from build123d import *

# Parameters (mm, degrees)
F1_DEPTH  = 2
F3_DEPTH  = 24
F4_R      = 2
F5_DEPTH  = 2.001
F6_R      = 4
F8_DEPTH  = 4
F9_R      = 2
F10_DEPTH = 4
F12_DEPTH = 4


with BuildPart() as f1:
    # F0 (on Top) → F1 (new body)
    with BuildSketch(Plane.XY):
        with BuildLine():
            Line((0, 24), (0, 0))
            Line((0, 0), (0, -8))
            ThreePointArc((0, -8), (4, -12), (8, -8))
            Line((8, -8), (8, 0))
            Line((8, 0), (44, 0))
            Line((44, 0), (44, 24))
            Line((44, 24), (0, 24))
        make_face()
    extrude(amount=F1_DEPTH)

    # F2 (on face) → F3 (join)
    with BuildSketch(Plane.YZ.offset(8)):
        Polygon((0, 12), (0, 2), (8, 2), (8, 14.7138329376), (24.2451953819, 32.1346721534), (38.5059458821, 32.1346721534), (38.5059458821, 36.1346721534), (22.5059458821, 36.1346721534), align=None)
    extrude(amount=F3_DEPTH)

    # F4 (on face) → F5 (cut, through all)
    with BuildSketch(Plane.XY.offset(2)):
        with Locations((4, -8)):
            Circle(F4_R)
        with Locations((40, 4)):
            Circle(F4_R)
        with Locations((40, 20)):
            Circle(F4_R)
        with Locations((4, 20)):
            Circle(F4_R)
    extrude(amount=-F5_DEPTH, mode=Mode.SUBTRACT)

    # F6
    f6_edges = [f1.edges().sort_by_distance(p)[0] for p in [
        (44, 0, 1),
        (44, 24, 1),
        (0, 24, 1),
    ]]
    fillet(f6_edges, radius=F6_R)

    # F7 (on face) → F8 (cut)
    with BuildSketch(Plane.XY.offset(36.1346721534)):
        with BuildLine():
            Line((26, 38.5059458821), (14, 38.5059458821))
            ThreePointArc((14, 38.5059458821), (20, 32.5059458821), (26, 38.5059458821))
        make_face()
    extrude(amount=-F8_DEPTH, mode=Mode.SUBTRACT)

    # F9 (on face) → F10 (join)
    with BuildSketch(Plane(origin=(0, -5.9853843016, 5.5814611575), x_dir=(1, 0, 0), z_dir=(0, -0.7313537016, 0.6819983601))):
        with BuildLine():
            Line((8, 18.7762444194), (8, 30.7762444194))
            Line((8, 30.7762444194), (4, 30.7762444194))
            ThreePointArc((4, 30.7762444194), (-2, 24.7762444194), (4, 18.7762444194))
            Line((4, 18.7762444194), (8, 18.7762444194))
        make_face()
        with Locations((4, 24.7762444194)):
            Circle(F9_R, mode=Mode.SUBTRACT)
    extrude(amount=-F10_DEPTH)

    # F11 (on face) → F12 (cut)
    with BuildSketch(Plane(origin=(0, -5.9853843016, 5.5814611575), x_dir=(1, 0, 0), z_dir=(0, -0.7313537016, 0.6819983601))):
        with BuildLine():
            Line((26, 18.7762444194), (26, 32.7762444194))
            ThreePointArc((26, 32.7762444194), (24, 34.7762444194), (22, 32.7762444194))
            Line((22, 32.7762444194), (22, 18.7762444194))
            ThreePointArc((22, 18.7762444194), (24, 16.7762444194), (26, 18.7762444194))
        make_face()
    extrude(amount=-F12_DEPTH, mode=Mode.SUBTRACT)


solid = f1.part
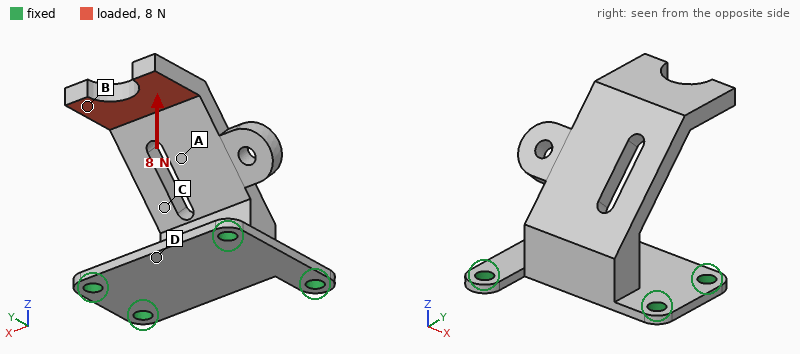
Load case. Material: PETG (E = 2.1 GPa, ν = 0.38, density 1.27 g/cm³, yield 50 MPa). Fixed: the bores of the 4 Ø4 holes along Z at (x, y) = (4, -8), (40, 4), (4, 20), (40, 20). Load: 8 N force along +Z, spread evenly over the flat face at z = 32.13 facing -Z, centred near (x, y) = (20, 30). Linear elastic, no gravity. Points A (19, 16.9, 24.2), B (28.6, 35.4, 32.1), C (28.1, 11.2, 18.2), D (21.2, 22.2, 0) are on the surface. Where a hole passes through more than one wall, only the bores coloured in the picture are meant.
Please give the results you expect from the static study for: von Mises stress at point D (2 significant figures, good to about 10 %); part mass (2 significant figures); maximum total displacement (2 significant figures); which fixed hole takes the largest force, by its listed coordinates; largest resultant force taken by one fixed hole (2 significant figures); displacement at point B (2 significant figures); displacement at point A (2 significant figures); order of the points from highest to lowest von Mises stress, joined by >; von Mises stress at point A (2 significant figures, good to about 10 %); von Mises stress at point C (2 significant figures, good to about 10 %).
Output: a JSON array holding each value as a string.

["1.3 MPa", "11 g", "0.89 mm", "(4, 20)", "8.4 N", "0.77 mm", "0.33 mm", "C > A > D > B", "2.3 MPa", "3.1 MPa"]
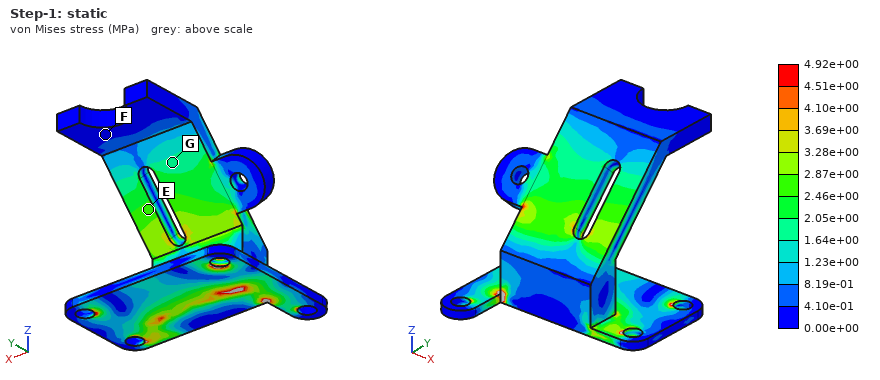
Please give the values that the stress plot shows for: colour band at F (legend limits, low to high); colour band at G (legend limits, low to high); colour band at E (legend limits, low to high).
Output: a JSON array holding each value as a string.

["0.00e+00 to 4.10e-01 MPa", "1.64e+00 to 2.05e+00 MPa", "2.46e+00 to 2.87e+00 MPa"]
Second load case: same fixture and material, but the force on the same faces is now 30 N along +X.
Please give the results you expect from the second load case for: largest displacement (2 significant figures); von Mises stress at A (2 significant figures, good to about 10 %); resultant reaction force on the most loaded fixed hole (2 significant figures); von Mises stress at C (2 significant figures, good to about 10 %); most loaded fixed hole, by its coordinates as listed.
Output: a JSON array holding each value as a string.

["0.79 mm", "3.7 MPa", "36 N", "3.5 MPa", "(40, 4)"]
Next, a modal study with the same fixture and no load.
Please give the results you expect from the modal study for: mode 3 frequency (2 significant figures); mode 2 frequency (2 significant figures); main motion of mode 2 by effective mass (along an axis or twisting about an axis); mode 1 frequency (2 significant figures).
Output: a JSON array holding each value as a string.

["1000 Hz", "660 Hz", "along X", "280 Hz"]
